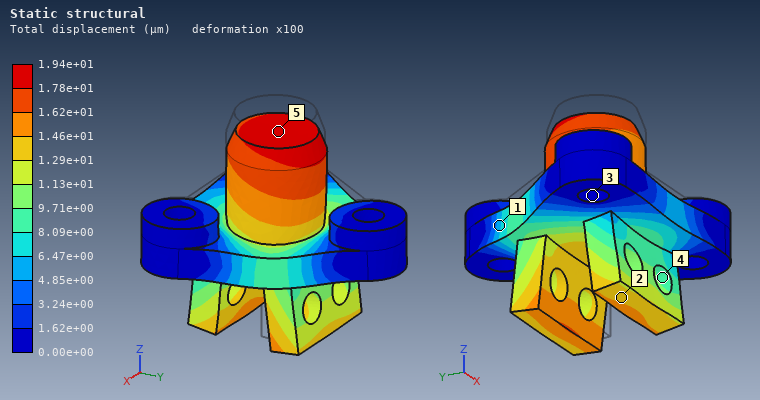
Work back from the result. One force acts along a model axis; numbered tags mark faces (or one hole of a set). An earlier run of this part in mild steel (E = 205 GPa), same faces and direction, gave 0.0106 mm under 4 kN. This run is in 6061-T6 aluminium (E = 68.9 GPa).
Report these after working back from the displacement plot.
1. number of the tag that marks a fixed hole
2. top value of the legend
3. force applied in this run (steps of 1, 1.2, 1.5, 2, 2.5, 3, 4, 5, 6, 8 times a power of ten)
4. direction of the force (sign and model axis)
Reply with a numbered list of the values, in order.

1. 3
2. 1.94e+01 µm
3. 2.5 kN
4. -Z
